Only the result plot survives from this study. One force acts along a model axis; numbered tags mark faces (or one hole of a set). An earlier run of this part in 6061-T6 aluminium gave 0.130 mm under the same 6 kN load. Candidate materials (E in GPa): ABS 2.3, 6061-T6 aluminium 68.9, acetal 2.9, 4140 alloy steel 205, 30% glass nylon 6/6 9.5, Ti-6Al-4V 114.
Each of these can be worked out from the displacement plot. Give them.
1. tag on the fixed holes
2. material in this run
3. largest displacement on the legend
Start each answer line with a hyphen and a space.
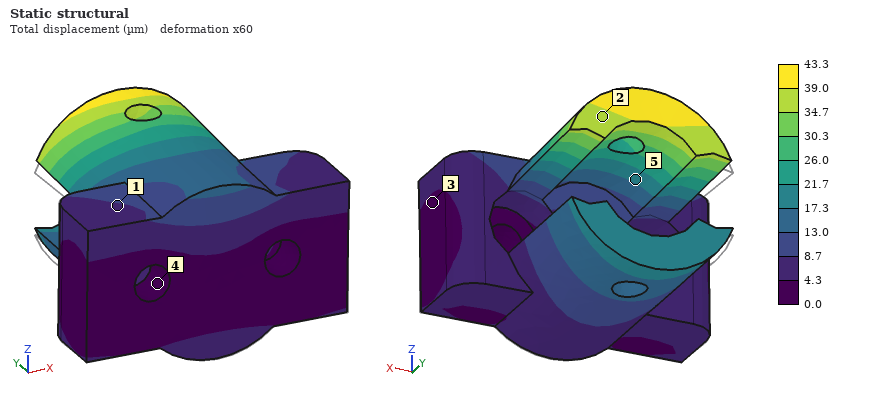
- 4
- 4140 alloy steel
- 43.3 µm
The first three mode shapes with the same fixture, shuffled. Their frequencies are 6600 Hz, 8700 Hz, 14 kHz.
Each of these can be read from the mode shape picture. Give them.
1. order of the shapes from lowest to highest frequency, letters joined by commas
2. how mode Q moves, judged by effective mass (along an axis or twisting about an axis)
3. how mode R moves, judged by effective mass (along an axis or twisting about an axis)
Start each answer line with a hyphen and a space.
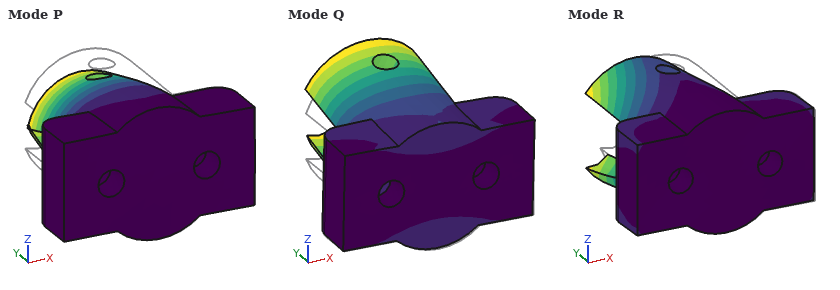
- Q, P, R
- along Z
- along X
